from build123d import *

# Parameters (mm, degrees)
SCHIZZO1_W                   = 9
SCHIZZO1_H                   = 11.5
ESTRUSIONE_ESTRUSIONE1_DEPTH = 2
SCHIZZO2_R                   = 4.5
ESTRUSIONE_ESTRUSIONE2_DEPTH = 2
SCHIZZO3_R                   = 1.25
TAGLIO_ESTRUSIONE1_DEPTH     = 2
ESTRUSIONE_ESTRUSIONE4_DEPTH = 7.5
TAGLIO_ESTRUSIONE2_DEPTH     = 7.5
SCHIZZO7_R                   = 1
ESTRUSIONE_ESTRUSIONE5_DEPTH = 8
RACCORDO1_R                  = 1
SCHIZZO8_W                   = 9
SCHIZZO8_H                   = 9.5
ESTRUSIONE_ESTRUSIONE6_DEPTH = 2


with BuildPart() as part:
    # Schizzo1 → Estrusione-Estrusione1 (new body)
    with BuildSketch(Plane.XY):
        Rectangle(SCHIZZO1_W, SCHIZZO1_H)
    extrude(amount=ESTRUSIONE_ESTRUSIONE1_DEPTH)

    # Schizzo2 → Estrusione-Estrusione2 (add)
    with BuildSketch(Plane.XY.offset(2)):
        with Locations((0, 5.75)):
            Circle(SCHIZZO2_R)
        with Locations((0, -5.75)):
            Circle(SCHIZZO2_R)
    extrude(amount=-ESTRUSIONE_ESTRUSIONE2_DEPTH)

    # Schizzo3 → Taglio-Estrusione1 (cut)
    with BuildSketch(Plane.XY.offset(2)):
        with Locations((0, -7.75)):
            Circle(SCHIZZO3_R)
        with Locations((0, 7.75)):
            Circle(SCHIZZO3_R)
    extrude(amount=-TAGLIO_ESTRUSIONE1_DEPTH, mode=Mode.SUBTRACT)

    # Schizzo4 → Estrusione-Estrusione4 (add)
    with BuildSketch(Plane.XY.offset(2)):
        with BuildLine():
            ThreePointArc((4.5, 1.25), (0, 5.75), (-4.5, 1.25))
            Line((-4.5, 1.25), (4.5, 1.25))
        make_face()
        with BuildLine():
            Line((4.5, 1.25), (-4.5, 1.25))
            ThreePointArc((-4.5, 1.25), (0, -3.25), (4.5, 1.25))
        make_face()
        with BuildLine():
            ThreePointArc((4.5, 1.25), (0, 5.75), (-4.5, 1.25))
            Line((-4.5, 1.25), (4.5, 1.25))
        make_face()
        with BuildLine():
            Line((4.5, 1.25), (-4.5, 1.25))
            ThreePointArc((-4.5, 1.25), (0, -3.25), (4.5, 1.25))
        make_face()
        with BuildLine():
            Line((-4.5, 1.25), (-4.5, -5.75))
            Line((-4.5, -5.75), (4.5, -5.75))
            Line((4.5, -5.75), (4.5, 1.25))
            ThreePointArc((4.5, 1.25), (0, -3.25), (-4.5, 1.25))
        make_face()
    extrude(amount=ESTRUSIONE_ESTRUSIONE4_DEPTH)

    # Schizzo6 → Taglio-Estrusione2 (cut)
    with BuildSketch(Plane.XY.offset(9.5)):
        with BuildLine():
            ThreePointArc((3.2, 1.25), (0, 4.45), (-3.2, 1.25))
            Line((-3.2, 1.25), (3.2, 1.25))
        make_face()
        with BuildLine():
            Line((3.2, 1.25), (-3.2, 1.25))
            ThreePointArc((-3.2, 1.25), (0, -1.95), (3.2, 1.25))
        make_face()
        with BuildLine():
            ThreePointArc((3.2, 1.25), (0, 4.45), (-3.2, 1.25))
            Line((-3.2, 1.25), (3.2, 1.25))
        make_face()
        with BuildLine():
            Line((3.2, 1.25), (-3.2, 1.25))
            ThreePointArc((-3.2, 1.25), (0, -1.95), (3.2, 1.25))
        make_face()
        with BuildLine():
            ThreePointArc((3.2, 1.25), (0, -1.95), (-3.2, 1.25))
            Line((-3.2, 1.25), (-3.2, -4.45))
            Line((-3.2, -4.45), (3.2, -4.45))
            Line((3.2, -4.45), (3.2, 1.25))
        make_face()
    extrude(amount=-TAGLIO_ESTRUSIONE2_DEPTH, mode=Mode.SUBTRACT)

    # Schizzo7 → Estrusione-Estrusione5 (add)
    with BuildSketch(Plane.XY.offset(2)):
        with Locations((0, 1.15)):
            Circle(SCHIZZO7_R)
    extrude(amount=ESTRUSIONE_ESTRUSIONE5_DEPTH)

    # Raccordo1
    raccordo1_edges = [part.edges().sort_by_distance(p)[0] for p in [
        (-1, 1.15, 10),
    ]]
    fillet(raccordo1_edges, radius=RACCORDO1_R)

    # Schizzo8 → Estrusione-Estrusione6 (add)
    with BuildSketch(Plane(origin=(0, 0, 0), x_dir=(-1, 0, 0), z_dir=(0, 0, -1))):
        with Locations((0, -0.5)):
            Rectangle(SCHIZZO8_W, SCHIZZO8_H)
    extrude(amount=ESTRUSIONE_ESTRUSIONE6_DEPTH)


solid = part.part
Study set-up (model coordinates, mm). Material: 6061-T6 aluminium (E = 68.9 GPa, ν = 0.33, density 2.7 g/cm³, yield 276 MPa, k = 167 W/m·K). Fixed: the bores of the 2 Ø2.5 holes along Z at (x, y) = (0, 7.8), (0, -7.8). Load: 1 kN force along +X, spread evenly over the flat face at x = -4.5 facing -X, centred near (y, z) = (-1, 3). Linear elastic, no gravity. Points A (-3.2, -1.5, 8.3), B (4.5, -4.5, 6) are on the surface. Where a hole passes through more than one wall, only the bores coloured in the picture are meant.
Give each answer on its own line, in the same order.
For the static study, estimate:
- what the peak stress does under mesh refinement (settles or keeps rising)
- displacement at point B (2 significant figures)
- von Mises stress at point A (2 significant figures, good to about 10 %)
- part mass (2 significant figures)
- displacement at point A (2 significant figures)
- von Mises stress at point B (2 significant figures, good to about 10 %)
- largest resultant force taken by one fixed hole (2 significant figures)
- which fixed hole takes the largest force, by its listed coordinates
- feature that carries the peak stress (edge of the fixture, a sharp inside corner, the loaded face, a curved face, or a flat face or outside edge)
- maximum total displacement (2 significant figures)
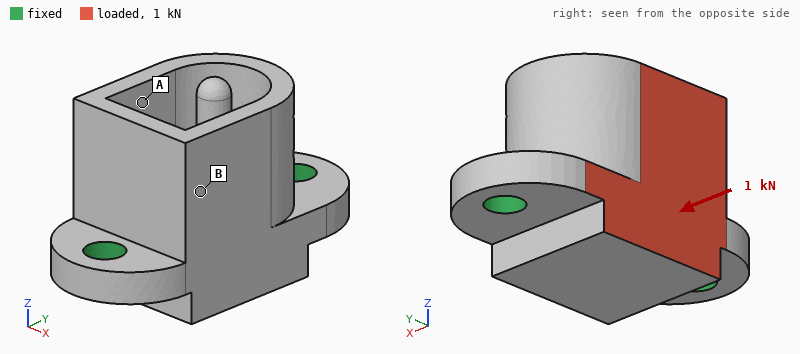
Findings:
keeps rising
31 µm
120 MPa
2.2 g
58 µm
27 MPa
600 N
(0, -7.8)
edge of the fixture
70 µm
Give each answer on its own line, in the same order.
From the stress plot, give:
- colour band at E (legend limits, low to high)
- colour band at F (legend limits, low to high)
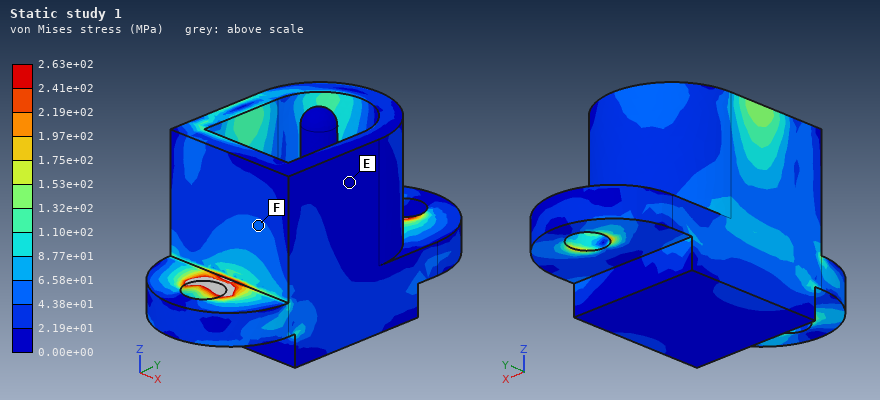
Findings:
0.00e+00 to 2.19e+01 MPa
4.38e+01 to 6.58e+01 MPa
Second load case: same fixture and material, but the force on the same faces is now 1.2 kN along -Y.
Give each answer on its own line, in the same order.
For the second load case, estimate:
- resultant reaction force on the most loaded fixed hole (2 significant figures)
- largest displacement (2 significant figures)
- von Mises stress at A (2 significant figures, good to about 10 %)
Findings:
730 N
22 µm
29 MPa
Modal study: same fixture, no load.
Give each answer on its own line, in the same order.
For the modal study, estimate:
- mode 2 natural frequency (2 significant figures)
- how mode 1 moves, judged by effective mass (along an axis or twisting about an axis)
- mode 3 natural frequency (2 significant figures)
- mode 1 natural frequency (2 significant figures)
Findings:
21 kHz
along X
22 kHz
17 kHz
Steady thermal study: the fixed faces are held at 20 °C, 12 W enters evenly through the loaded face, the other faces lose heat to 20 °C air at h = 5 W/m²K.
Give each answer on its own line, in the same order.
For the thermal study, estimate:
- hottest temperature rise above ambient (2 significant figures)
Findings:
17 K
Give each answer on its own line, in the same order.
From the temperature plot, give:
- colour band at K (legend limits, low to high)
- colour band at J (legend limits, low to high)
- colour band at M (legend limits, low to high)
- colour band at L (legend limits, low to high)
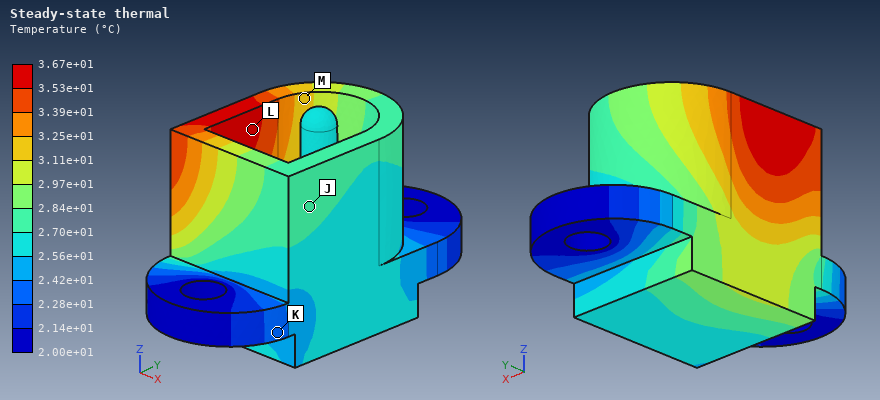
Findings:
2.28e+01 to 2.42e+01 °C
2.70e+01 to 2.84e+01 °C
3.11e+01 to 3.25e+01 °C
3.53e+01 to 3.67e+01 °C
